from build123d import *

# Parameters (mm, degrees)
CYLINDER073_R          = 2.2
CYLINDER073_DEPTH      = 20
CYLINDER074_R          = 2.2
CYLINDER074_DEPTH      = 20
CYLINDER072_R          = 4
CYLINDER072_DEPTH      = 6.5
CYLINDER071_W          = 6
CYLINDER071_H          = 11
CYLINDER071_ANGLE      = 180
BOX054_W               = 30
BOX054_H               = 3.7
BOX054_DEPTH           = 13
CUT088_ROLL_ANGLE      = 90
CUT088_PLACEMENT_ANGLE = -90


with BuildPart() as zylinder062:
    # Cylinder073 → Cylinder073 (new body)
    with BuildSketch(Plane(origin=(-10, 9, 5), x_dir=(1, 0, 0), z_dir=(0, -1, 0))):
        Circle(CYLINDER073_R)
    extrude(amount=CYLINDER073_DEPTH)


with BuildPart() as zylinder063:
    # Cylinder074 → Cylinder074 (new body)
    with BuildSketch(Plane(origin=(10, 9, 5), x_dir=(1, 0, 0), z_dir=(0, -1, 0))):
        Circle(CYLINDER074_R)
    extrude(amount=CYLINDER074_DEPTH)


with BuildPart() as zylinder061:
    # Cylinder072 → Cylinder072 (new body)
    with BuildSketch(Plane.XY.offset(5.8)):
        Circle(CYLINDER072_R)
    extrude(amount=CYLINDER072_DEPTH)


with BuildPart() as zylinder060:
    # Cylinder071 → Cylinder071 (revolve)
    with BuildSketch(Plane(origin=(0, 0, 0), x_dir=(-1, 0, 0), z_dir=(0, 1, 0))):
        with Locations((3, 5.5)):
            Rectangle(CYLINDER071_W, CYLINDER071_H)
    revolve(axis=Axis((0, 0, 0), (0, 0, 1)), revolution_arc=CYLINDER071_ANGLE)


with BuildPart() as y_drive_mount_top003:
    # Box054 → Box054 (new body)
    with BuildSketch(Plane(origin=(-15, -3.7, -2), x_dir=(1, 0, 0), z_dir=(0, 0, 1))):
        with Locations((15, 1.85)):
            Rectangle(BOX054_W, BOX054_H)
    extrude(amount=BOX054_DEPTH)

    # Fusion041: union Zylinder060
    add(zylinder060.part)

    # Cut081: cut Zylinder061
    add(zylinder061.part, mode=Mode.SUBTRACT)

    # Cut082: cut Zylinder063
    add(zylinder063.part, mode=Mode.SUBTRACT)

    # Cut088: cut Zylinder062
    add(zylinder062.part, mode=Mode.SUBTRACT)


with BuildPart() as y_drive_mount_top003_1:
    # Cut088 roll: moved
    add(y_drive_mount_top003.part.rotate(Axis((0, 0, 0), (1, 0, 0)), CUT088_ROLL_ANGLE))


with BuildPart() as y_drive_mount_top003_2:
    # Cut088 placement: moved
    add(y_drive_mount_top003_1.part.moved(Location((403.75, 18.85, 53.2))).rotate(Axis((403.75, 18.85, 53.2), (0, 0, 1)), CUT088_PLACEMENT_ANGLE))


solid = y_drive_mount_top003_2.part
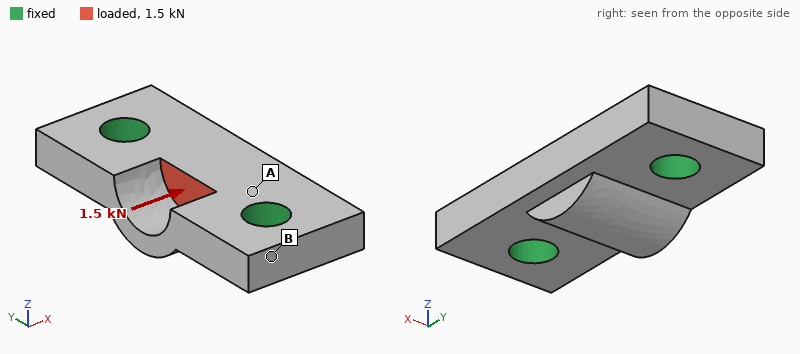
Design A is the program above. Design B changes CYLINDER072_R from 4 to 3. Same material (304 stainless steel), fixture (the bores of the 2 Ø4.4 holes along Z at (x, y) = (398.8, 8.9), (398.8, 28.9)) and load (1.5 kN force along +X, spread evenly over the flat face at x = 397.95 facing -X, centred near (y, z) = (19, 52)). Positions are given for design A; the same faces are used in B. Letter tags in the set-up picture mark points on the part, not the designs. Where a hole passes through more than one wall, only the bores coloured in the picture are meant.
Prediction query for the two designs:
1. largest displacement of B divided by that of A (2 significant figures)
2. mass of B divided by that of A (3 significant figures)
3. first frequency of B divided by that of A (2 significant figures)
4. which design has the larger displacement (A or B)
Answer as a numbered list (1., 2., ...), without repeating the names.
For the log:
1. 1.2
2. 1.04
3. 1.00
4. B
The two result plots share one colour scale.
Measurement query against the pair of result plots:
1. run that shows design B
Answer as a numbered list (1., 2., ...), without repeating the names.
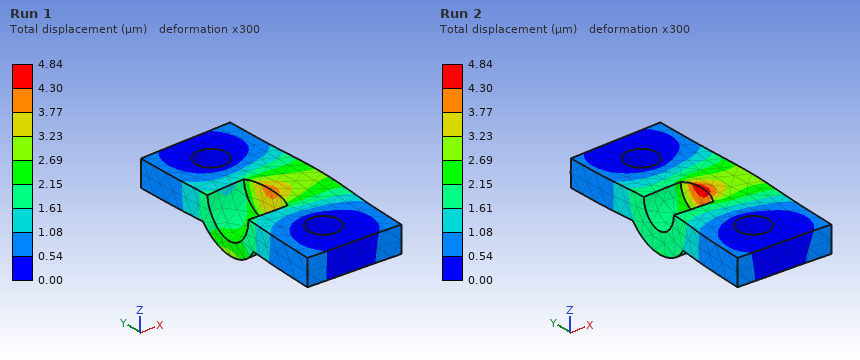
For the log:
1. Run 2
